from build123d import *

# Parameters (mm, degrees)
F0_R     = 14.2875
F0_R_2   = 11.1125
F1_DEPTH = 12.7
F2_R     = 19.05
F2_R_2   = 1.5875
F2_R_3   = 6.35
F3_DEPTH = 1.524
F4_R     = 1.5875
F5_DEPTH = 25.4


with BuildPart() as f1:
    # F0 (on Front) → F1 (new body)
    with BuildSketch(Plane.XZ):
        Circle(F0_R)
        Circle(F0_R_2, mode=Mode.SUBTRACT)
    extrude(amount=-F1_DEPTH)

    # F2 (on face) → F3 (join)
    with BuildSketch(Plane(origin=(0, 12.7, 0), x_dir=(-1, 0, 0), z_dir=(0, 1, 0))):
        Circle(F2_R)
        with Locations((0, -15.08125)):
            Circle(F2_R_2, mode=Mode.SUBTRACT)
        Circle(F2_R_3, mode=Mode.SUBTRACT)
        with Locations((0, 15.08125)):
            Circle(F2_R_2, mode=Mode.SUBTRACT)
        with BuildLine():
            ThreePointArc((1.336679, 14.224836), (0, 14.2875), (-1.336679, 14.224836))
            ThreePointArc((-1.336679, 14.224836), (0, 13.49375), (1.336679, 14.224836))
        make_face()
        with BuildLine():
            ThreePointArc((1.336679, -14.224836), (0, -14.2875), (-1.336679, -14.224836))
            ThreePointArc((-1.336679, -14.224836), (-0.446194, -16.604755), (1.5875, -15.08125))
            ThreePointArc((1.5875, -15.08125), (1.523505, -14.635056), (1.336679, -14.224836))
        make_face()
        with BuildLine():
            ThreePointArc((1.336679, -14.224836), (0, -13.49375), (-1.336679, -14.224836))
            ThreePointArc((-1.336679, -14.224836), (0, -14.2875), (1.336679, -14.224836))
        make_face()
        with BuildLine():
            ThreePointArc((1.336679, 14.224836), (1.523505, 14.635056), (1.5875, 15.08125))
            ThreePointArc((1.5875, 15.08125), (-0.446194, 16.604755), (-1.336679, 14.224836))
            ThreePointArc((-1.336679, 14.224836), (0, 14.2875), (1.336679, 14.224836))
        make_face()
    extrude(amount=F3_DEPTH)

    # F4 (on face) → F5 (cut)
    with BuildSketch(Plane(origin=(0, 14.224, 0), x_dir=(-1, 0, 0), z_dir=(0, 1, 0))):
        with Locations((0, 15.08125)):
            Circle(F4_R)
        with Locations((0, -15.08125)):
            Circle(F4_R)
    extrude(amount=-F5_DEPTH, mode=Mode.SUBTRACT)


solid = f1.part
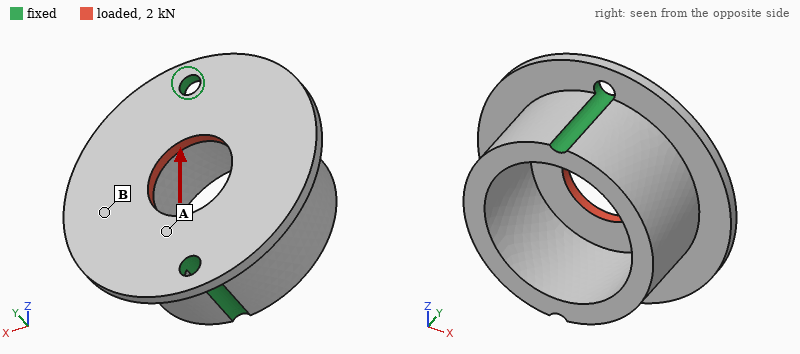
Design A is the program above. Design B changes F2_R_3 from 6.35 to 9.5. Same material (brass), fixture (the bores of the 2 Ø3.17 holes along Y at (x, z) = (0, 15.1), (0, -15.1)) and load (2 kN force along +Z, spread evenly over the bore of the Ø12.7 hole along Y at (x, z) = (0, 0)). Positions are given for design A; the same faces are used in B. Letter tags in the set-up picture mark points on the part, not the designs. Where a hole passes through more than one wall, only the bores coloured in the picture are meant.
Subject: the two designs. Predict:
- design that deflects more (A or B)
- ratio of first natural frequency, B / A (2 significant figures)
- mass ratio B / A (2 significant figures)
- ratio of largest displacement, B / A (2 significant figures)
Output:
B
0.99
0.95
1.1
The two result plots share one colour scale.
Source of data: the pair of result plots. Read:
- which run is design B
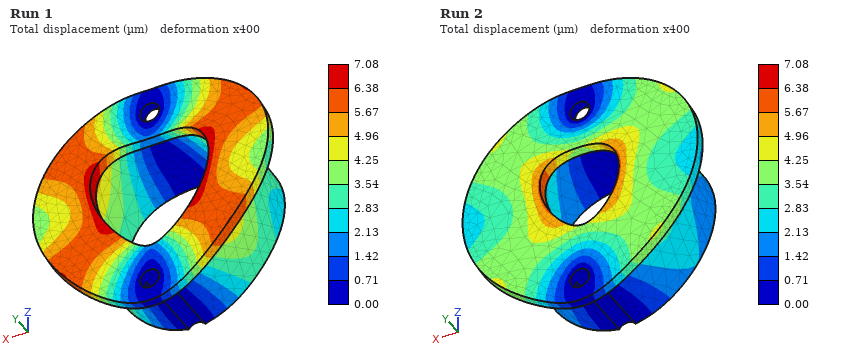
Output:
Run 1
